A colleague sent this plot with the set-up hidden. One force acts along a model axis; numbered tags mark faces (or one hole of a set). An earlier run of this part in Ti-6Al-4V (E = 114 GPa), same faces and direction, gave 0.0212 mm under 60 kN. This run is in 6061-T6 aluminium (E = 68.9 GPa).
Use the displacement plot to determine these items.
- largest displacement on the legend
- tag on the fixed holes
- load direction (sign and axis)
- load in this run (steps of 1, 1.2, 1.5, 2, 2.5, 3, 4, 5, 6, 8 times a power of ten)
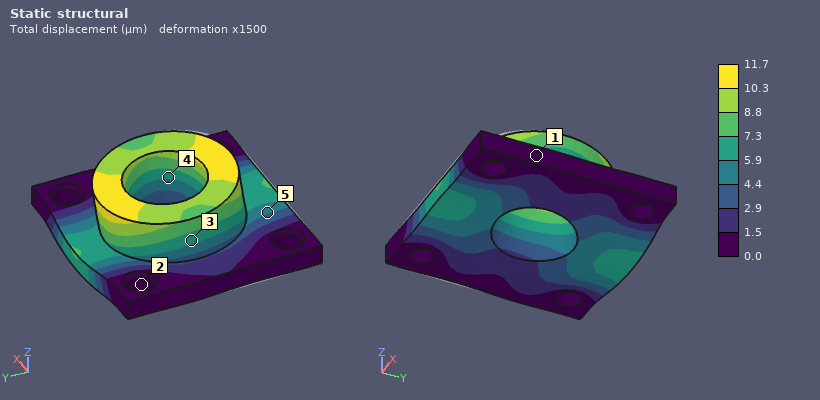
11.7 µm
2
+Y
20 kN
